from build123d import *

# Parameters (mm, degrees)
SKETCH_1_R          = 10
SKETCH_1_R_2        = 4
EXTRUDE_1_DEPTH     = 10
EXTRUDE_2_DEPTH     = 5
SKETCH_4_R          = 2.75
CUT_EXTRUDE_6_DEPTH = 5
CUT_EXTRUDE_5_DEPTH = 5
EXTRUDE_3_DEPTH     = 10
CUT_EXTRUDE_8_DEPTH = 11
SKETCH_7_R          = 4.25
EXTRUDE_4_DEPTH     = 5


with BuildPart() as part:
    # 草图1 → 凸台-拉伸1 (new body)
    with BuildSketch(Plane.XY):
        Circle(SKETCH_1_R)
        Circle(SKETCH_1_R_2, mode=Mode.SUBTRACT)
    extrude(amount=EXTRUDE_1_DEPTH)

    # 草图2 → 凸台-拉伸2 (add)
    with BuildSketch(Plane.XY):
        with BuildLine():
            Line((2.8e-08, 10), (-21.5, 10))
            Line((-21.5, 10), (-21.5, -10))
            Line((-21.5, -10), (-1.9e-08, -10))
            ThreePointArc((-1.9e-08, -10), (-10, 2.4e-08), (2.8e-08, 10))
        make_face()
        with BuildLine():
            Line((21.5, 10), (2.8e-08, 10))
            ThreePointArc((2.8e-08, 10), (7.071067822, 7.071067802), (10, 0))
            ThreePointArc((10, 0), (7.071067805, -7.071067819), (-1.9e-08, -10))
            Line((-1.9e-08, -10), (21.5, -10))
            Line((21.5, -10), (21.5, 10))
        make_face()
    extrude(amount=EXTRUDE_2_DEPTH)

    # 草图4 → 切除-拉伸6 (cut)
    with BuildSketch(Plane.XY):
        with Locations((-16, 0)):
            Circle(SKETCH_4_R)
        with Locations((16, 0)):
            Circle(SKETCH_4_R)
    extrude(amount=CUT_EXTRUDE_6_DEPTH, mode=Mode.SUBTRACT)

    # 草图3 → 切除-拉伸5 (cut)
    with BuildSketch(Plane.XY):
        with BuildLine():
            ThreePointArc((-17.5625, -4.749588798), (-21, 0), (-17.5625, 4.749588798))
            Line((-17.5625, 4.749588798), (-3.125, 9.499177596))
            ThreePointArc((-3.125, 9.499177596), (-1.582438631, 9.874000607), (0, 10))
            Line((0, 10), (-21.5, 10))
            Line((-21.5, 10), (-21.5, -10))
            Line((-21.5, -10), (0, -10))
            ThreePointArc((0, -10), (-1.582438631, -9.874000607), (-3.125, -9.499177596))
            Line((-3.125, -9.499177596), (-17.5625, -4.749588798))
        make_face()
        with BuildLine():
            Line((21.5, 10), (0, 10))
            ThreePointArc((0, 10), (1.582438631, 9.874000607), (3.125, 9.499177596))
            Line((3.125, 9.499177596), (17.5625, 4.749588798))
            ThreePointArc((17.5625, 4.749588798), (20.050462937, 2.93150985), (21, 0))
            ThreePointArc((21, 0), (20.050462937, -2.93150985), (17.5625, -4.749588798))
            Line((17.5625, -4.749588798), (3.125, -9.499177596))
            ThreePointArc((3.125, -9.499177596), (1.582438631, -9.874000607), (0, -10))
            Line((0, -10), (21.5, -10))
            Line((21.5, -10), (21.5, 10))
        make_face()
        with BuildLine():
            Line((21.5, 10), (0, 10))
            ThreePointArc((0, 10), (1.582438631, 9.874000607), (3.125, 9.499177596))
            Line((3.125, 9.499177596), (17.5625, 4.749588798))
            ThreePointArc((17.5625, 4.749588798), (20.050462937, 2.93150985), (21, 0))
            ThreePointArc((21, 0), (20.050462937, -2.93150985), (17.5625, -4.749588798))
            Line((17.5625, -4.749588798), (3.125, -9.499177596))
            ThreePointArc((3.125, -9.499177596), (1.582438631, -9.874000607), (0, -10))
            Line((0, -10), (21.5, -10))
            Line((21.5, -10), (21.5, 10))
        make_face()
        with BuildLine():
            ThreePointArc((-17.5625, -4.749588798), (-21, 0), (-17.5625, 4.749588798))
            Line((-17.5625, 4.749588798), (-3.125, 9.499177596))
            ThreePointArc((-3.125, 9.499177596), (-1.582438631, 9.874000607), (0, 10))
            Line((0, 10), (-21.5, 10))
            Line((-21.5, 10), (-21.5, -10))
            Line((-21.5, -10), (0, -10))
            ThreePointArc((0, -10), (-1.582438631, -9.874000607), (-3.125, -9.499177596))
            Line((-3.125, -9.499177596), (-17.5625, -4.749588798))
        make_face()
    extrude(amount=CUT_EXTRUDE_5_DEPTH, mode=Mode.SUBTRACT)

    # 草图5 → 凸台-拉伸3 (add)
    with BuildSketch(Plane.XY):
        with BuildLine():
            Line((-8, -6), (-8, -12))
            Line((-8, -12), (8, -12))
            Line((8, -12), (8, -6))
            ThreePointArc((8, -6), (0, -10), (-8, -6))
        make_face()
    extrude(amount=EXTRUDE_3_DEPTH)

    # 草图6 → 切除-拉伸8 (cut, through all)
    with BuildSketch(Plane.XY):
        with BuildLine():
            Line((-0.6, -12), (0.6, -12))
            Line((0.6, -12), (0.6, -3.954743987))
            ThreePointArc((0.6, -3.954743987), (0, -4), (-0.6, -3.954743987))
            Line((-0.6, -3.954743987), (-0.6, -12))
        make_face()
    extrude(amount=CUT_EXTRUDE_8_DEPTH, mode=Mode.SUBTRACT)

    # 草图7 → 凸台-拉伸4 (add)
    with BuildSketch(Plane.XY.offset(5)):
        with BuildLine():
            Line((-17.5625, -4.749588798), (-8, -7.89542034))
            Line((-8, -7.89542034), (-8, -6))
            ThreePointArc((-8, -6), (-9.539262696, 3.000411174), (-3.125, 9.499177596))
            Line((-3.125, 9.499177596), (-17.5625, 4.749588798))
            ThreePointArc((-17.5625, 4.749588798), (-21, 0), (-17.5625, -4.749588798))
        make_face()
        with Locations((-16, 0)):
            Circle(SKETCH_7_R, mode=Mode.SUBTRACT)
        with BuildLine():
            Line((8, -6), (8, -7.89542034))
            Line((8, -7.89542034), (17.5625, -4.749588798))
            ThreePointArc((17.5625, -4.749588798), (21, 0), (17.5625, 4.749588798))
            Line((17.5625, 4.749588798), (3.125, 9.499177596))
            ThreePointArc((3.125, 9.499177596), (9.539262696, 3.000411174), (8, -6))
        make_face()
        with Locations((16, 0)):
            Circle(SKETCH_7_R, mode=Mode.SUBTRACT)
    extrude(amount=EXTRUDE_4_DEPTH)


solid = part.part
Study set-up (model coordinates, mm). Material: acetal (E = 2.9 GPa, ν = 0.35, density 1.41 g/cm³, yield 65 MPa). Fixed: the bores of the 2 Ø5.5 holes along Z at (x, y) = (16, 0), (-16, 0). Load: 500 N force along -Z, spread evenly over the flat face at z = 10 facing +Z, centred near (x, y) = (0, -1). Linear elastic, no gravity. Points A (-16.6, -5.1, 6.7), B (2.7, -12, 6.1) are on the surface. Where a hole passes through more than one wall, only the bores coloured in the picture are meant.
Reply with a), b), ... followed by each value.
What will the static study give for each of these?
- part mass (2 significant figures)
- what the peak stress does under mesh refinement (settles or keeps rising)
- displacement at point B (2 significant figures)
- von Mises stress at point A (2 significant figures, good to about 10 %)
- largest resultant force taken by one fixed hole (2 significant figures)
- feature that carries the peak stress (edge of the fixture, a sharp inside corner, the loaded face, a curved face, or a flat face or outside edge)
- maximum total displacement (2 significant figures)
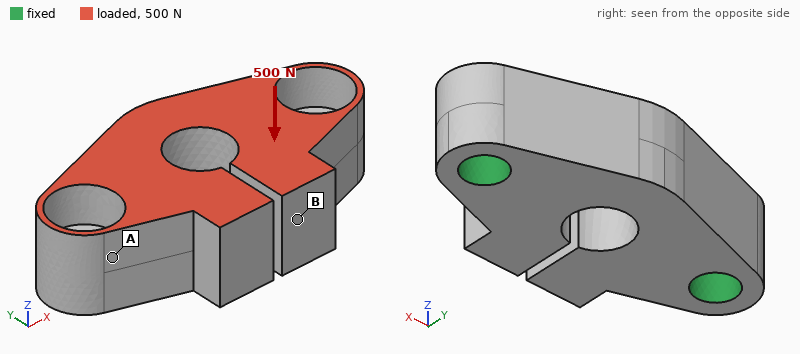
a) 6.9 g
b) keeps rising
c) 0.12 mm
d) 5.2 MPa
e) 260 N
f) edge of the fixture
g) 0.14 mm
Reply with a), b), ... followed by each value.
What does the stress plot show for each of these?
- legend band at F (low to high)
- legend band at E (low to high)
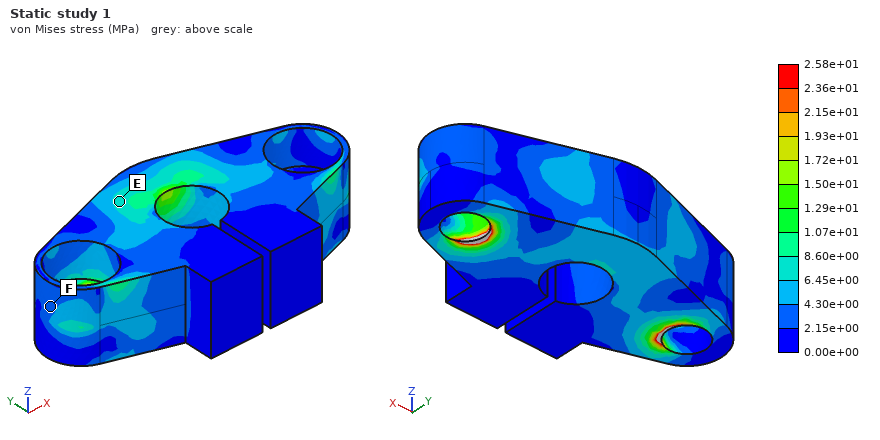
a) 2.15e+00 to 4.30e+00 MPa
b) 6.45e+00 to 8.60e+00 MPa
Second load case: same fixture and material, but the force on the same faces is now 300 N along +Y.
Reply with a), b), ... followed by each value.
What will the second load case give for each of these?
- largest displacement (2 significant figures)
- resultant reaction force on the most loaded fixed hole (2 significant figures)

a) 0.12 mm
b) 170 N
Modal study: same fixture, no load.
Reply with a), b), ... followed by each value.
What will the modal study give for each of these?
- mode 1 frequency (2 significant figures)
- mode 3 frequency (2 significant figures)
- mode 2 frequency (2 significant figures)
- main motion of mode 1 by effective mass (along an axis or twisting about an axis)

a) 4600 Hz
b) 5300 Hz
c) 5000 Hz
d) along Z
